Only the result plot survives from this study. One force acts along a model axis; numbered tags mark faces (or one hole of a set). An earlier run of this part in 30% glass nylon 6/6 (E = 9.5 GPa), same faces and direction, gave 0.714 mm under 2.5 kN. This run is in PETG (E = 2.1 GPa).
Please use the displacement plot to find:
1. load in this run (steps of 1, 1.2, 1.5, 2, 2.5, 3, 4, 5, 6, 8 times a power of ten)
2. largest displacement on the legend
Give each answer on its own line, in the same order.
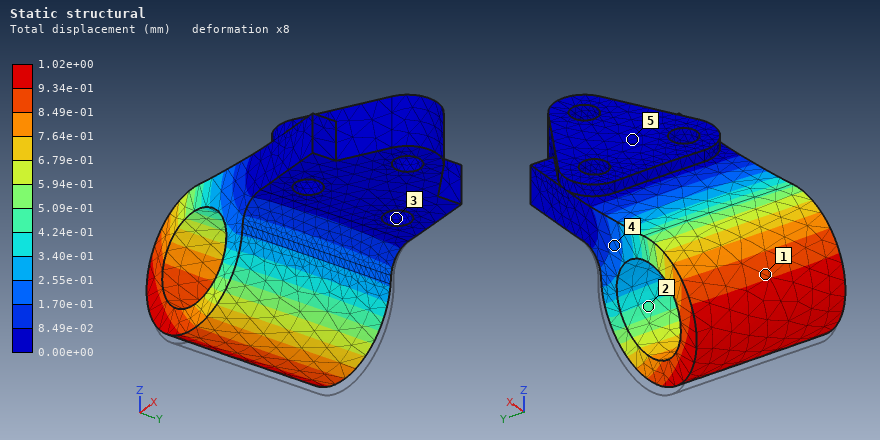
800 N
1.02e+00 mm
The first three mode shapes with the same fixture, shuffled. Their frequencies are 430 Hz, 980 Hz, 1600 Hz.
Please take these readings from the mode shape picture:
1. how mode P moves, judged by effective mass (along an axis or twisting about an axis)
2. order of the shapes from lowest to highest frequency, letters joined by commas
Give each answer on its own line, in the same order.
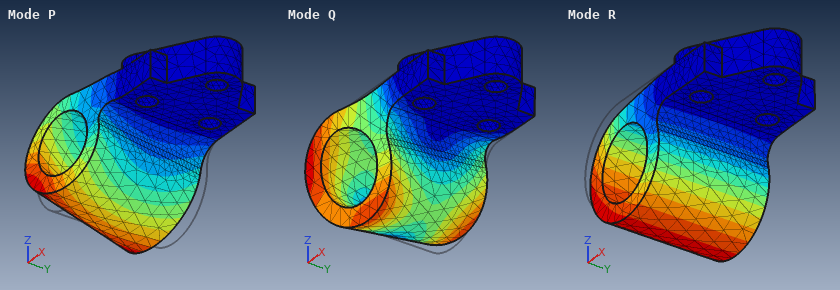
along Y
R, P, Q
